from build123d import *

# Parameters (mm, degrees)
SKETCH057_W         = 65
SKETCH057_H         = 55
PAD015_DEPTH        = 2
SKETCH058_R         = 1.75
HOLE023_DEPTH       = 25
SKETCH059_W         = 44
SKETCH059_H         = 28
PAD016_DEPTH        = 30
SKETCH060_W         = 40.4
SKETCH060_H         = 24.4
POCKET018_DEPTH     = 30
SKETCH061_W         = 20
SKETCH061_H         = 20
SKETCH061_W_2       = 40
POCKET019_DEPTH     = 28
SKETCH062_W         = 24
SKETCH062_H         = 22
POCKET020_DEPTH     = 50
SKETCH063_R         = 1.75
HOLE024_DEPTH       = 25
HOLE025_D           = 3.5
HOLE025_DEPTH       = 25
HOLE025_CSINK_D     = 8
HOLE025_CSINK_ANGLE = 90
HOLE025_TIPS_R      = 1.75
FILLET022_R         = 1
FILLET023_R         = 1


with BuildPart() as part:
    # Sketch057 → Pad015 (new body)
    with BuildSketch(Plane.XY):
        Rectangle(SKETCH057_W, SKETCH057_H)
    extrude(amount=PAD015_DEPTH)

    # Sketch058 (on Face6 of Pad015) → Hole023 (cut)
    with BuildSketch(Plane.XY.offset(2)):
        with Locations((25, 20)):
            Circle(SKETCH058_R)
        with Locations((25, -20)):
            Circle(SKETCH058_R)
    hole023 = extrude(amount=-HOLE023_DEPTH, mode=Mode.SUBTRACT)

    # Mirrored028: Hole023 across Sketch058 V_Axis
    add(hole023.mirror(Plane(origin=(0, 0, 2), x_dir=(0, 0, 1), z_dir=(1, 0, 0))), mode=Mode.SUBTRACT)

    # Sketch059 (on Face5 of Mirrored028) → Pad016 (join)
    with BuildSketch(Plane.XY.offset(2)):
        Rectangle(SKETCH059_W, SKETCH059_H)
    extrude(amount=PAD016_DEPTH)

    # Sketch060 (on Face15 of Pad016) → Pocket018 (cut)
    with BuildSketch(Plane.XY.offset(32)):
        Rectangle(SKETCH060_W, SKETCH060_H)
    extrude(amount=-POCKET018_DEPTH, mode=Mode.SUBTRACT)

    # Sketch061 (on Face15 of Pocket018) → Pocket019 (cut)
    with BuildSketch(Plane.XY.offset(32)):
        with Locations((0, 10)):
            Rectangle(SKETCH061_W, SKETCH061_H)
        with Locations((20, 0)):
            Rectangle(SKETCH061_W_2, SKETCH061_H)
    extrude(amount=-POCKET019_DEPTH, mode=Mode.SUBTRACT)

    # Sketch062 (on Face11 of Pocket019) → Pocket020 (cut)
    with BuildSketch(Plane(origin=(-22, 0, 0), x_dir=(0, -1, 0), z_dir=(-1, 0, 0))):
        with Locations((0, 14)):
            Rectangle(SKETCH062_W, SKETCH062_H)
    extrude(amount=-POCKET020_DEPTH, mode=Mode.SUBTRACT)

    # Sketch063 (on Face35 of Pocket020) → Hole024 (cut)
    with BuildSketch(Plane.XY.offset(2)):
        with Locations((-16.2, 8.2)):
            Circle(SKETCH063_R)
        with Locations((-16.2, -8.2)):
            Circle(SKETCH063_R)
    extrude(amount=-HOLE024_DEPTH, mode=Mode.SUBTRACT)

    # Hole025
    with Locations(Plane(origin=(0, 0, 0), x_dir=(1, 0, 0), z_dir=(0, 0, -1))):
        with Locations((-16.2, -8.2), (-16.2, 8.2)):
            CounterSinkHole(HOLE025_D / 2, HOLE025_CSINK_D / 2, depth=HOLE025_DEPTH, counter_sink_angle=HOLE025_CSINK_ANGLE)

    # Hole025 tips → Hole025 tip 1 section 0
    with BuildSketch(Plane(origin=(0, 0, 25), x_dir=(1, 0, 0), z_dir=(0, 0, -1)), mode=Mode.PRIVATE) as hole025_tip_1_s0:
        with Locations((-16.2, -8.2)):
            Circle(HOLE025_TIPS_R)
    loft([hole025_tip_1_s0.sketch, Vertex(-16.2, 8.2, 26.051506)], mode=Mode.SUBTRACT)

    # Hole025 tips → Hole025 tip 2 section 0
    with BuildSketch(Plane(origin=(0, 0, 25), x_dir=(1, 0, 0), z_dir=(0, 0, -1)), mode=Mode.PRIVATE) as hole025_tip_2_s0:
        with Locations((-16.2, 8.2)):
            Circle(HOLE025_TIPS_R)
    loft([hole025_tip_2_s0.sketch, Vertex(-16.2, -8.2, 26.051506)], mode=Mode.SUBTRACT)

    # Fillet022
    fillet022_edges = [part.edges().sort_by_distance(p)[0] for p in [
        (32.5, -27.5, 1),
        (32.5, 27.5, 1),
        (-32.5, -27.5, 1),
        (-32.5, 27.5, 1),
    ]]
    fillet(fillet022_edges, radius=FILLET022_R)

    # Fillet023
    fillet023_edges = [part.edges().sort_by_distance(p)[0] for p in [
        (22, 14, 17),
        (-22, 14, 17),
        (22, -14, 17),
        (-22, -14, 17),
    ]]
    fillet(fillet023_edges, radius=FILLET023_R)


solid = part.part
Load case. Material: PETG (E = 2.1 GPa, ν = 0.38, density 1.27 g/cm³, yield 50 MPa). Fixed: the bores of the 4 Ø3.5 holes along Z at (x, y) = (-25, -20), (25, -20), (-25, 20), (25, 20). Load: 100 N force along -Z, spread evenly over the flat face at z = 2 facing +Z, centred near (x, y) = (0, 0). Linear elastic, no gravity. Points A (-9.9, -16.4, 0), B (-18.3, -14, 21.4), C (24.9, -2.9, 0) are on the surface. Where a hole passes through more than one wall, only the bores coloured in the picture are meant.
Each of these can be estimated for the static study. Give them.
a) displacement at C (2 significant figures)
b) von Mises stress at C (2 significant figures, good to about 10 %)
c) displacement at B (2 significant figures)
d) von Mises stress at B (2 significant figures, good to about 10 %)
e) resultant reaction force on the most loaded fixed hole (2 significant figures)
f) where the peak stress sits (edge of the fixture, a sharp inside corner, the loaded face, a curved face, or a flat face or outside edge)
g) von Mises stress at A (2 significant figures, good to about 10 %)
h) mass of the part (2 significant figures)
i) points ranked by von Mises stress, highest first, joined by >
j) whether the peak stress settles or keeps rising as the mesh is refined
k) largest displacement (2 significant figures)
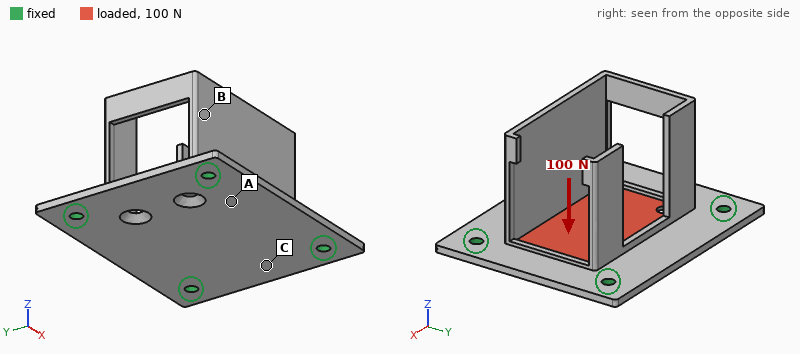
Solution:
0.24 mm
4.3 MPa
0.24 mm
1.4 MPa
30 N
edge of the fixture
2.3 MPa
14 g
C > A > B
keeps rising
0.99 mm
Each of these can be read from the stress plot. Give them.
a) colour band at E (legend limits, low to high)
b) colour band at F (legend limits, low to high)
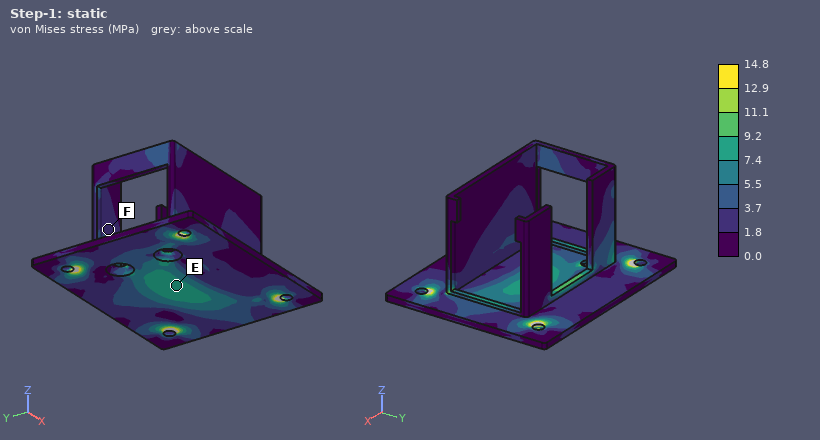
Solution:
7.4 to 9.2 MPa
1.8 to 3.7 MPa
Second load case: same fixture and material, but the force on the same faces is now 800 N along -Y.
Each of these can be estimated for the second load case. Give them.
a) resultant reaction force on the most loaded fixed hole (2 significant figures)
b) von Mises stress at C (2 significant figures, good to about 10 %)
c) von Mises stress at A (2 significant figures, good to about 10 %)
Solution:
240 N
2.5 MPa
3.2 MPa
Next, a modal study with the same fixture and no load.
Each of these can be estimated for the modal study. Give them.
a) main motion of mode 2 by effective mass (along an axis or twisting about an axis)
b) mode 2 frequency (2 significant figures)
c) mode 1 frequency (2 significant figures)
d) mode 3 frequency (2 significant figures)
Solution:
along Y
450 Hz
380 Hz
650 Hz
